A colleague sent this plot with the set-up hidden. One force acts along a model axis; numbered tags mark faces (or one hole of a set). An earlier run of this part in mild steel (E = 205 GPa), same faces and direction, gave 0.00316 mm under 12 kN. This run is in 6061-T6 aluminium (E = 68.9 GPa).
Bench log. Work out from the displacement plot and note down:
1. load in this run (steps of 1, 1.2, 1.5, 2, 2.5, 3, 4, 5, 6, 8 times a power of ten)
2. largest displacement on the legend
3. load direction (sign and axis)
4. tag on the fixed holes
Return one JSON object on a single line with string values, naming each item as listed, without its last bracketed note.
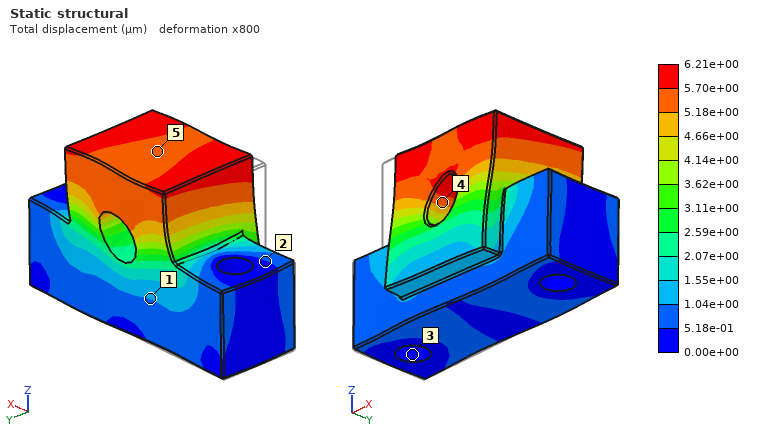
{"load in this run": "8 kN", "largest displacement on the legend": "6.21e+00 µm", "load direction": "+X", "tag on the fixed holes": "3"}
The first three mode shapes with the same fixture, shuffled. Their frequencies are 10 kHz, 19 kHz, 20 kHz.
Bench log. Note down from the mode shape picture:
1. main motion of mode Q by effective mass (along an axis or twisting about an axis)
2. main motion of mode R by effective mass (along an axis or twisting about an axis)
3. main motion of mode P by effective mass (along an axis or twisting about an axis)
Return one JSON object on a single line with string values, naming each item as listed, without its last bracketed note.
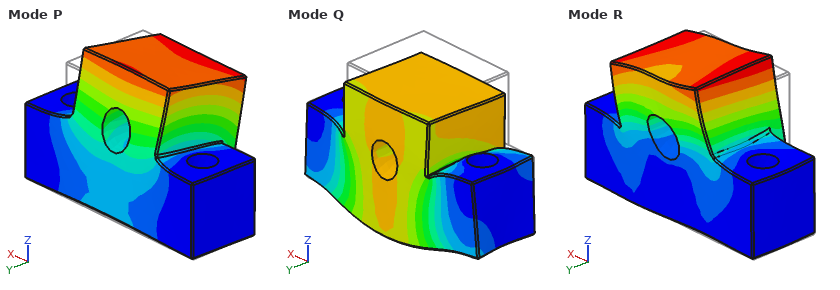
{"main motion of mode Q by effective mass": "along Z", "main motion of mode R by effective mass": "along X", "main motion of mode P by effective mass": "along Y"}
